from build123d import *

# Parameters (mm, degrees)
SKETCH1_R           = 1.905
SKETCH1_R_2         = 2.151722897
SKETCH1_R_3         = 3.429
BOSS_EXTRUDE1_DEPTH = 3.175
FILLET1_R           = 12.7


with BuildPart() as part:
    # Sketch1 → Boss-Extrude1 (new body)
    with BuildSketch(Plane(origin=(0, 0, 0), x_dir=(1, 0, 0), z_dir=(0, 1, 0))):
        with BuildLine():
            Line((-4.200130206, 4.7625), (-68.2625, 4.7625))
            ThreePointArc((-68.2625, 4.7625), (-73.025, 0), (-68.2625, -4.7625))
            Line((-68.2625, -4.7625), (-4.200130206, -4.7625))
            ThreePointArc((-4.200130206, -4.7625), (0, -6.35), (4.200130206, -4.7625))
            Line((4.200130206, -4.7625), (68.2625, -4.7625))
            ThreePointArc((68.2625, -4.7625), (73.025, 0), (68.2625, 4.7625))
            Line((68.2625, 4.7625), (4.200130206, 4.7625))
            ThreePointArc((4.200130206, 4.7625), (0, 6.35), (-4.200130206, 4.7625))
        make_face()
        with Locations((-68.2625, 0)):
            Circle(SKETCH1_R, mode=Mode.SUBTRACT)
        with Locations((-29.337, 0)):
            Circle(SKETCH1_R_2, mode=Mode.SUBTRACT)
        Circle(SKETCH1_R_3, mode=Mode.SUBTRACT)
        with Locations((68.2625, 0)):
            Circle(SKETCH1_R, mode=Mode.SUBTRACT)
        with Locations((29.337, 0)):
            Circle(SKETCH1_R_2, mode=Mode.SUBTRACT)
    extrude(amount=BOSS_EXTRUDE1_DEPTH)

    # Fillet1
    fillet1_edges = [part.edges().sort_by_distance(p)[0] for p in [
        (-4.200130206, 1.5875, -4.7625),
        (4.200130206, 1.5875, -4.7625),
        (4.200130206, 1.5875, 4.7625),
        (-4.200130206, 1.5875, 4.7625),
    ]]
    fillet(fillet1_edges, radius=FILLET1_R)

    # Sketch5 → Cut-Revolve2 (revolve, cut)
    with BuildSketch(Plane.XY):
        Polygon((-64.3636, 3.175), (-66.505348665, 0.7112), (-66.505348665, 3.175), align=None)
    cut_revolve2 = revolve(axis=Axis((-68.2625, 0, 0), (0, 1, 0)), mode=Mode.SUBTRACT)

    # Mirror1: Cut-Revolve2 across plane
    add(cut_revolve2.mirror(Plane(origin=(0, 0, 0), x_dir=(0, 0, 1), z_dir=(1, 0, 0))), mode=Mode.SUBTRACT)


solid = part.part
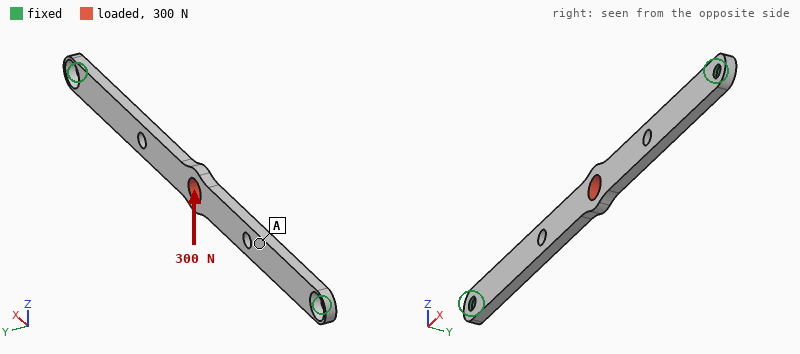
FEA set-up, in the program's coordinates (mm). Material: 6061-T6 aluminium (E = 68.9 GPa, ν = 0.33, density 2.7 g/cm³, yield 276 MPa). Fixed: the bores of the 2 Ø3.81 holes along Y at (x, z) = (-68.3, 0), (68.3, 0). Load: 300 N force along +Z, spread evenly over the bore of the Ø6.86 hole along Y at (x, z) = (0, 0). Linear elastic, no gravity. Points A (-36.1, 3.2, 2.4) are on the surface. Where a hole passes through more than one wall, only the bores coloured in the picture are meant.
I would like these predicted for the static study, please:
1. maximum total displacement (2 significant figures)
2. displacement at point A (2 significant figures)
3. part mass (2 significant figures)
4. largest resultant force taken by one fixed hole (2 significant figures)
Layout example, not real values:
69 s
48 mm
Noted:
0.34 mm
0.18 mm
11 g
150 N
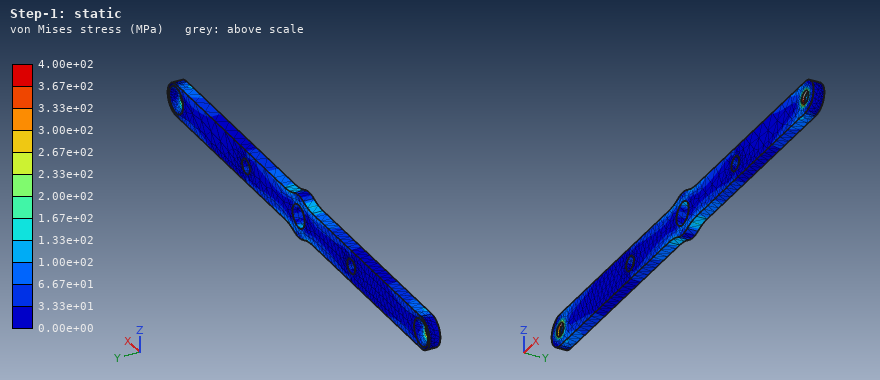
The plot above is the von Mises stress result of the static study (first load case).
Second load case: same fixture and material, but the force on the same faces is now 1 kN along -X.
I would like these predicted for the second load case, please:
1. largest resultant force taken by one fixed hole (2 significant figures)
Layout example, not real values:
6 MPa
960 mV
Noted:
500 N
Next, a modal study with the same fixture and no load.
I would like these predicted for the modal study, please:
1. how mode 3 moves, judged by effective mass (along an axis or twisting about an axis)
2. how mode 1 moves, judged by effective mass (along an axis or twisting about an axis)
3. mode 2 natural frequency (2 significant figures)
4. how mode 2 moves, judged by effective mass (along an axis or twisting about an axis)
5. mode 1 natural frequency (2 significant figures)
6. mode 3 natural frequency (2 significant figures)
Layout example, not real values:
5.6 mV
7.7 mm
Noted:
along Z
along Y
2100 Hz
twisting about Z
780 Hz
2200 Hz
